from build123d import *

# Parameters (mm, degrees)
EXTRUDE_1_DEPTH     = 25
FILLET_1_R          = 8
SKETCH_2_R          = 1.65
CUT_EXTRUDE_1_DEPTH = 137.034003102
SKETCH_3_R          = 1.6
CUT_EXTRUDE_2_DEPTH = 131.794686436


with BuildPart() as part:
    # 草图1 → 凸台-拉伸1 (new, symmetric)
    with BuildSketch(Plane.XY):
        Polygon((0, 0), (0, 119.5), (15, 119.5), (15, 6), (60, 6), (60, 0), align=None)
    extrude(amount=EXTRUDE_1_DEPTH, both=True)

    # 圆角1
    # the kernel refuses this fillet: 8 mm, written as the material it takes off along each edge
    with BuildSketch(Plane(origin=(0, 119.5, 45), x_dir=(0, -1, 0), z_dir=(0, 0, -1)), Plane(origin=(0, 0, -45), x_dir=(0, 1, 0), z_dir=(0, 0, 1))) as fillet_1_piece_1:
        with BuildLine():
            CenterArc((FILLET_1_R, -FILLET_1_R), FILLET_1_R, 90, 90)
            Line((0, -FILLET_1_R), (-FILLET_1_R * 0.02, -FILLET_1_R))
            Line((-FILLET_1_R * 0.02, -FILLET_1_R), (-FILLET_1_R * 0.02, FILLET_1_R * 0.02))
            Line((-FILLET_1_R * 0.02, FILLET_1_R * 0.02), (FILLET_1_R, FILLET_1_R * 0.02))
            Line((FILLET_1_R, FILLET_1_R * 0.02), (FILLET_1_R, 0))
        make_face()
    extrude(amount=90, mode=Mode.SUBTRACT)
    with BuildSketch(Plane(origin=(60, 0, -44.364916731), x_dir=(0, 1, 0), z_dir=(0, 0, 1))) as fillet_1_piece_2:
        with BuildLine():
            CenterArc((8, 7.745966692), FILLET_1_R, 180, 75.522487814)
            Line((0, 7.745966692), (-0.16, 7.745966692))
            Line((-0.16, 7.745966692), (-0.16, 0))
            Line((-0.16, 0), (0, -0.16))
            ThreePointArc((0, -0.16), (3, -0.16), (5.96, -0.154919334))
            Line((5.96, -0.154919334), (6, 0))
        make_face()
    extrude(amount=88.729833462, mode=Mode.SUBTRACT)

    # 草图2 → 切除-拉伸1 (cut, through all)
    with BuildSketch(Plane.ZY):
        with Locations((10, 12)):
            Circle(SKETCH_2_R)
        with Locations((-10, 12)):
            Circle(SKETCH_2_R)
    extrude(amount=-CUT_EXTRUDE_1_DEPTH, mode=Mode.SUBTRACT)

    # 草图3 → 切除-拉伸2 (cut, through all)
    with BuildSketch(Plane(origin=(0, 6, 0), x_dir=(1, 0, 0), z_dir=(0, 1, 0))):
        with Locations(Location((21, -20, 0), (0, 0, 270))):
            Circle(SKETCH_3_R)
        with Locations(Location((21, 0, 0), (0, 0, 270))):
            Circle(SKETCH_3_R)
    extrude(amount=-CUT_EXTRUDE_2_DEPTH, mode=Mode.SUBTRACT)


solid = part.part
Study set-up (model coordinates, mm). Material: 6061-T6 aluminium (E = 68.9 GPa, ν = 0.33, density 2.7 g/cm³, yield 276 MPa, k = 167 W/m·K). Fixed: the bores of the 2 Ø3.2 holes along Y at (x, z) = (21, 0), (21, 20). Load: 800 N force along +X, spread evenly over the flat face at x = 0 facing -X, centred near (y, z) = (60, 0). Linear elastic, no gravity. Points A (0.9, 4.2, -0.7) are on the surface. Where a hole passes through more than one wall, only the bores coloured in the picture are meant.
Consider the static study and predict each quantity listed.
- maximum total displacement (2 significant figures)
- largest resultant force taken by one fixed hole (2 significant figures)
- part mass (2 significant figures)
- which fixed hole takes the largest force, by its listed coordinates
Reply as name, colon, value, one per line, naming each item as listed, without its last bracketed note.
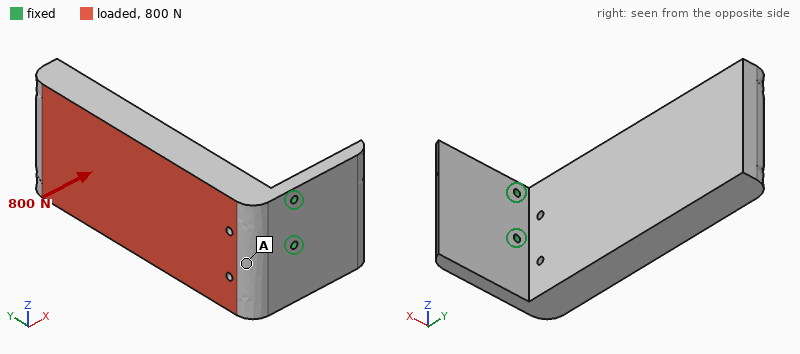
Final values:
maximum total displacement: 1.2 mm
largest resultant force taken by one fixed hole: 780 N
part mass: 270 g
which fixed hole takes the largest force, by its listed coordinates: (21, 0)
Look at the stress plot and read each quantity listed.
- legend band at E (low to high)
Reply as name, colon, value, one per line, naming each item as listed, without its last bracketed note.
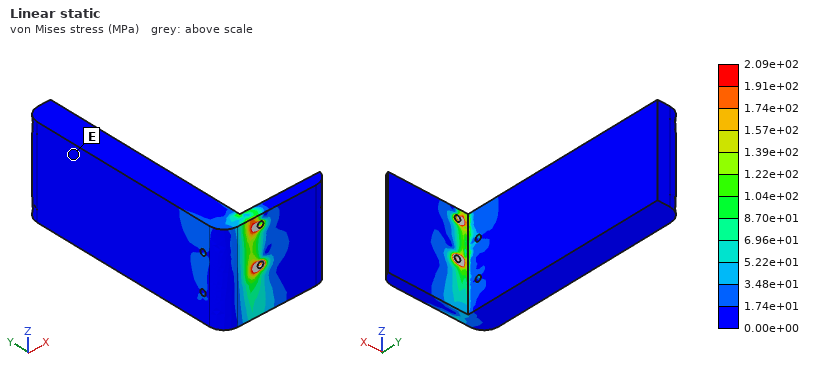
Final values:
legend band at E: 0.00e+00 to 1.74e+01 MPa
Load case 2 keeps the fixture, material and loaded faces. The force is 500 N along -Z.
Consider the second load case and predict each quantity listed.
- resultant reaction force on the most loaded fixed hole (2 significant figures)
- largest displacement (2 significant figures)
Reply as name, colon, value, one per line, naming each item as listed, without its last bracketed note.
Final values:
resultant reaction force on the most loaded fixed hole: 1.3 kN
largest displacement: 0.13 mm
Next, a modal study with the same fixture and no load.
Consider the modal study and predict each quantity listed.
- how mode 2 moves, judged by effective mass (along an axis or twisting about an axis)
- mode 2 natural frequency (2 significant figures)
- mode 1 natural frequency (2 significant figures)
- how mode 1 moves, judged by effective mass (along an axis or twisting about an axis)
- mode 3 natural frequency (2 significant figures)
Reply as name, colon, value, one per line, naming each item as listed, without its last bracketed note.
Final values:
how mode 2 moves, judged by effective mass: along Z
mode 2 natural frequency: 780 Hz
mode 1 natural frequency: 320 Hz
how mode 1 moves, judged by effective mass: along X
mode 3 natural frequency: 3000 Hz
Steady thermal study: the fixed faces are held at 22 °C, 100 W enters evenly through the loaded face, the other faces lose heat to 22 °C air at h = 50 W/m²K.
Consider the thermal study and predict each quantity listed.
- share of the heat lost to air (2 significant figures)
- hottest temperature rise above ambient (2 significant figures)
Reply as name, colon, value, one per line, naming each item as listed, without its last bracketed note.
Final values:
share of the heat lost to air: 27 %
hottest temperature rise above ambient: 55 K
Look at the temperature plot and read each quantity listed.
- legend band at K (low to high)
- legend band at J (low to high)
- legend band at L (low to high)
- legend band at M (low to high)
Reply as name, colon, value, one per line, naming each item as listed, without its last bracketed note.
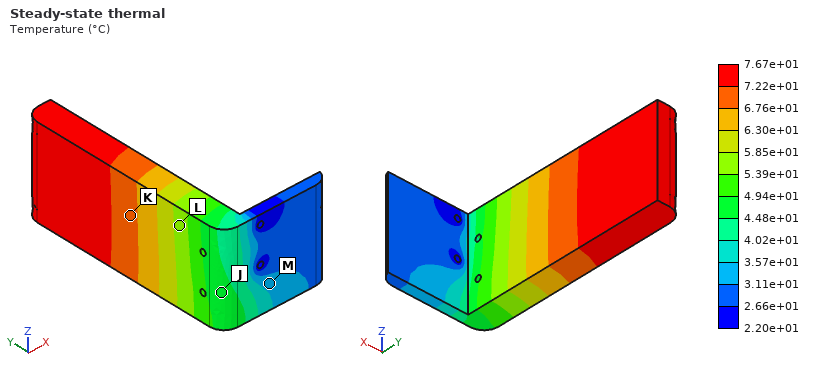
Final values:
legend band at K: 6.76e+01 to 7.22e+01 °C
legend band at J: 4.48e+01 to 4.94e+01 °C
legend band at L: 5.39e+01 to 5.85e+01 °C
legend band at M: 3.11e+01 to 3.57e+01 °C
